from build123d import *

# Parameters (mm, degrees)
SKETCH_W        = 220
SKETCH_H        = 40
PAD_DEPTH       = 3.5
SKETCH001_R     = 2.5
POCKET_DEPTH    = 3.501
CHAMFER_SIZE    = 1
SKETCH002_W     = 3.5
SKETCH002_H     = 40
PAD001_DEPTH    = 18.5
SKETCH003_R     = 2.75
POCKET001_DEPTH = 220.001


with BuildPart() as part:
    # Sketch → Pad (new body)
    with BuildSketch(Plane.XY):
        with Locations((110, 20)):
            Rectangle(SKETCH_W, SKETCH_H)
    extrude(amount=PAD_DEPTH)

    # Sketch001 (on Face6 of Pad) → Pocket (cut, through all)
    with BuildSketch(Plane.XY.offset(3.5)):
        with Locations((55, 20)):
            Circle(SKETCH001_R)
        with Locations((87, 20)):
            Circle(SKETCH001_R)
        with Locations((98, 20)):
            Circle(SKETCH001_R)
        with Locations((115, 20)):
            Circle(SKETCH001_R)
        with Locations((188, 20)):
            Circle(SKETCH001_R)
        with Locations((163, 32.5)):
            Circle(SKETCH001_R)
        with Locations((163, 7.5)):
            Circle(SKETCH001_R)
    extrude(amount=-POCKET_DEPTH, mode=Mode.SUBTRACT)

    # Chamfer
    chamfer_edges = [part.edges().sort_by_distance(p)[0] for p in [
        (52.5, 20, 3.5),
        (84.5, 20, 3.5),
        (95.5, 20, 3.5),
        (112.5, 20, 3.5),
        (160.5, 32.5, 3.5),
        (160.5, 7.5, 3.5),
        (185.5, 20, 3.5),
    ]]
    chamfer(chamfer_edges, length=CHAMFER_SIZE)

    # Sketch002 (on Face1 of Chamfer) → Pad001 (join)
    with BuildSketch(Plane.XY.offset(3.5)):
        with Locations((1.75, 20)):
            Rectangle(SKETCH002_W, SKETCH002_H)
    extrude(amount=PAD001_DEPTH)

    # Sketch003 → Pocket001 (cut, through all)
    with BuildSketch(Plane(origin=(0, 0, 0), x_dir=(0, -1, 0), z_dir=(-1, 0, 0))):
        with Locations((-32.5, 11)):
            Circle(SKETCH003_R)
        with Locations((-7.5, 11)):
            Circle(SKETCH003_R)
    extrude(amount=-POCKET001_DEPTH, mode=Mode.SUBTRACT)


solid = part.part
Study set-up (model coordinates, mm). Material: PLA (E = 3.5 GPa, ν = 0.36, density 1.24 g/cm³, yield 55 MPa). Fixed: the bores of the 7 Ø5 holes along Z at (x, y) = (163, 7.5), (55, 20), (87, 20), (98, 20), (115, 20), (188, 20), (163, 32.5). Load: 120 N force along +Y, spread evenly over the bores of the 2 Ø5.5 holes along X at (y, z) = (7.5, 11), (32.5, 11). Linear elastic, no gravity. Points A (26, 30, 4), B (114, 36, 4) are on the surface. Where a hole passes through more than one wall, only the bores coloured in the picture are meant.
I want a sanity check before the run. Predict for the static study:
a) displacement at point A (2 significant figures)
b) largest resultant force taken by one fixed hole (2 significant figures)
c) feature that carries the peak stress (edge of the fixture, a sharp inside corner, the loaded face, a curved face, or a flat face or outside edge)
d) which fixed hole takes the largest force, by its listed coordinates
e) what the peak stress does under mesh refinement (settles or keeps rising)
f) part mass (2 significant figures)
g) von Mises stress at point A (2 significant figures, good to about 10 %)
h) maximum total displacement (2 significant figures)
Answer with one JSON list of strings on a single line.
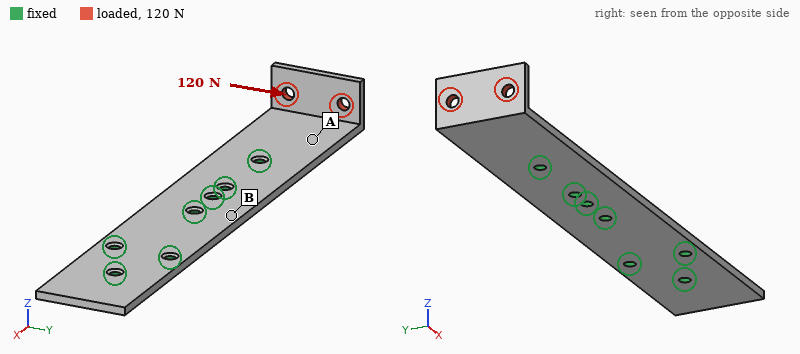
["0.52 mm", "250 N", "edge of the fixture", "(55, 20)", "keeps rising", "41 g", "13 MPa", "2.5 mm"]
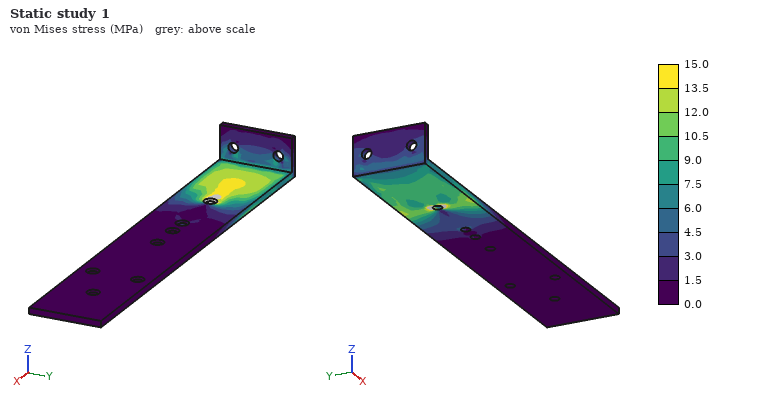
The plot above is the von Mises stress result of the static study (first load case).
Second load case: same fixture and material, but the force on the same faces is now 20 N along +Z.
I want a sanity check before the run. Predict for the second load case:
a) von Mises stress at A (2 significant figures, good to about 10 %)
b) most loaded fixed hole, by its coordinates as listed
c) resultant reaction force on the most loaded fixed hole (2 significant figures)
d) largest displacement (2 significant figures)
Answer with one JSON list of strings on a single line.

["5.7 MPa", "(55, 20)", "38 N", "2.5 mm"]
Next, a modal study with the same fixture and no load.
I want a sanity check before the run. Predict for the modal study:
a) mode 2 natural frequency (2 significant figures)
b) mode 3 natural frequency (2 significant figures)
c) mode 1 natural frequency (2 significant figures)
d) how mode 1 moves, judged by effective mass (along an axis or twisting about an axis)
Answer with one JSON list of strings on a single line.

["500 Hz", "850 Hz", "200 Hz", "along Z"]
